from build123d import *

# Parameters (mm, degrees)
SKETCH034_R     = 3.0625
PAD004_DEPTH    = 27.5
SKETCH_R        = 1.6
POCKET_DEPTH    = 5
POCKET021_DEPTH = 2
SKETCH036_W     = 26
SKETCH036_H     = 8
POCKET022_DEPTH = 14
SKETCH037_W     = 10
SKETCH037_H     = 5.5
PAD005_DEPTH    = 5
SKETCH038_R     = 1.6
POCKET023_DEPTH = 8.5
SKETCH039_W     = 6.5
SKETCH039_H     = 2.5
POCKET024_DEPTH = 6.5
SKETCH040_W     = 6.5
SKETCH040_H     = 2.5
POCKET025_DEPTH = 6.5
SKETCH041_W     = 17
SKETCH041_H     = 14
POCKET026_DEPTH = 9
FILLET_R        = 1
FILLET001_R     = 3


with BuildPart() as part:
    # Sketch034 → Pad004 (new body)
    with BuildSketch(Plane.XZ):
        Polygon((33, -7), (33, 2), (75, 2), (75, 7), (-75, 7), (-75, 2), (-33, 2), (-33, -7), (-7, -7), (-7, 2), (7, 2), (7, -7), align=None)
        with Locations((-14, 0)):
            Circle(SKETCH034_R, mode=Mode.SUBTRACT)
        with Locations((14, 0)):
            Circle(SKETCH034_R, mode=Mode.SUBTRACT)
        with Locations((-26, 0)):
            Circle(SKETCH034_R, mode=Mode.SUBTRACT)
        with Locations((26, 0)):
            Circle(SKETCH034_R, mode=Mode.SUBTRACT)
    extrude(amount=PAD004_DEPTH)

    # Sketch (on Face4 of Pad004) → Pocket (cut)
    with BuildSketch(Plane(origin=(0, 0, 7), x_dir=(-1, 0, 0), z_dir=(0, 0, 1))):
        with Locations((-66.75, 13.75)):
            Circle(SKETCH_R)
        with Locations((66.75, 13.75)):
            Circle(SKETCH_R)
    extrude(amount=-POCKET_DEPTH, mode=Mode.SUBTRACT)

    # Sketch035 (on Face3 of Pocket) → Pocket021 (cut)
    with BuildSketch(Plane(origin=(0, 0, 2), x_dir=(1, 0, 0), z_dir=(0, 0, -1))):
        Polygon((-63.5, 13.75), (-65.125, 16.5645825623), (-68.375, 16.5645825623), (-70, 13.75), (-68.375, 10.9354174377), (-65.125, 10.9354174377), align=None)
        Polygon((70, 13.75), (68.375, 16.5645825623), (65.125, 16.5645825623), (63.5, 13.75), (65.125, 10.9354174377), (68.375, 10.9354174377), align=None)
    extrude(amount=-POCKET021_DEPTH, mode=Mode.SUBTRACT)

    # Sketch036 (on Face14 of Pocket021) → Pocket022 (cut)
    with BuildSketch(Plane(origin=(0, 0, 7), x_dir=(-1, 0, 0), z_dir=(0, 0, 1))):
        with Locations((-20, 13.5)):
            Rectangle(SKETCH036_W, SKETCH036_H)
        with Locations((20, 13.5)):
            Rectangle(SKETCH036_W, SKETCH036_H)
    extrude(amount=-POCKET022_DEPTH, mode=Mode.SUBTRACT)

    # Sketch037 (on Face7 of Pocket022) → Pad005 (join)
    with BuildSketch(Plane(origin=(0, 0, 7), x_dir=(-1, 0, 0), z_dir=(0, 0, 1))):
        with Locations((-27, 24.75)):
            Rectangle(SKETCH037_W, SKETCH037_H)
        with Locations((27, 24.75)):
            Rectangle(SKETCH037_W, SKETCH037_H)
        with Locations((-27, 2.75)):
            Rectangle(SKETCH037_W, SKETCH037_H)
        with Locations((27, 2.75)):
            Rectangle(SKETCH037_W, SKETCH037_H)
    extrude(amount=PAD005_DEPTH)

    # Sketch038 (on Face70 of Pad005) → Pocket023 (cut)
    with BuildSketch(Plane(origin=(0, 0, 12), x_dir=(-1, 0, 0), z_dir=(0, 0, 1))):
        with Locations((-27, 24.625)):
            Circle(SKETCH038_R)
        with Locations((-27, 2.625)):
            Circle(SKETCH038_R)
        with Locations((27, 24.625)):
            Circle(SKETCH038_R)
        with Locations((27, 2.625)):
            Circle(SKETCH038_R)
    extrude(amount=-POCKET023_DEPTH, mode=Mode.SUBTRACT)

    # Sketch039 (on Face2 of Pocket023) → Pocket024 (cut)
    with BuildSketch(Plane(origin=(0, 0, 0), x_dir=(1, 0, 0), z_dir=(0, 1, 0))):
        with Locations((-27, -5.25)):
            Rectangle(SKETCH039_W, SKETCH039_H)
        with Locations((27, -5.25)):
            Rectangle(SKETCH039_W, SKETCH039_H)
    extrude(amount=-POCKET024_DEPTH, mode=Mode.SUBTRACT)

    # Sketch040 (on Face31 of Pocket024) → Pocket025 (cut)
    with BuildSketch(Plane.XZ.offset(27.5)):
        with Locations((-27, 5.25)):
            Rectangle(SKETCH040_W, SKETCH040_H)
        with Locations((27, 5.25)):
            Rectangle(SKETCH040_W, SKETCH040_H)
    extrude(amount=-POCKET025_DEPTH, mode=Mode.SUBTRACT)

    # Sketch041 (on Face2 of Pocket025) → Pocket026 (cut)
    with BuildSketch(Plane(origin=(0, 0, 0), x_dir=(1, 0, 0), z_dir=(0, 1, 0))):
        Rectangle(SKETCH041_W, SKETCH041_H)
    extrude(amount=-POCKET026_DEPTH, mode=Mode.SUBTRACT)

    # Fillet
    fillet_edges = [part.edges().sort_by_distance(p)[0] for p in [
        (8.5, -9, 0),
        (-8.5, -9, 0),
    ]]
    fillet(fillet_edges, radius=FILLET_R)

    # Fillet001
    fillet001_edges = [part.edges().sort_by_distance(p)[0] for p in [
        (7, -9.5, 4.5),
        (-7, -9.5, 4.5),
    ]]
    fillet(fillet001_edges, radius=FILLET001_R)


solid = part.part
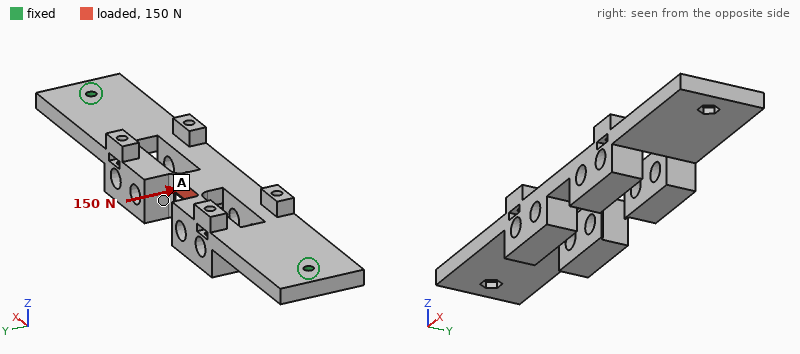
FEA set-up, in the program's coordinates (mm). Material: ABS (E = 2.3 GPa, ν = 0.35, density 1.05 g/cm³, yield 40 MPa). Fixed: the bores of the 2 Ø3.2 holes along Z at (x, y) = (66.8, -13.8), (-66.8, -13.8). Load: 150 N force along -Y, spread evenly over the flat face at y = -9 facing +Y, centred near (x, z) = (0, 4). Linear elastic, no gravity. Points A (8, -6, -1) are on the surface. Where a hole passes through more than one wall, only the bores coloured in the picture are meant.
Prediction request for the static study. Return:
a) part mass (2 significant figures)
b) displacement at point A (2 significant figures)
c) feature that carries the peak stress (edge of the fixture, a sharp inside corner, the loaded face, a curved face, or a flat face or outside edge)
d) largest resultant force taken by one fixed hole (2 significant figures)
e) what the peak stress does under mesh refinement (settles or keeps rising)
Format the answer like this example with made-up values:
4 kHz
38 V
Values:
26 g
0.93 mm
edge of the fixture
180 N
keeps rising
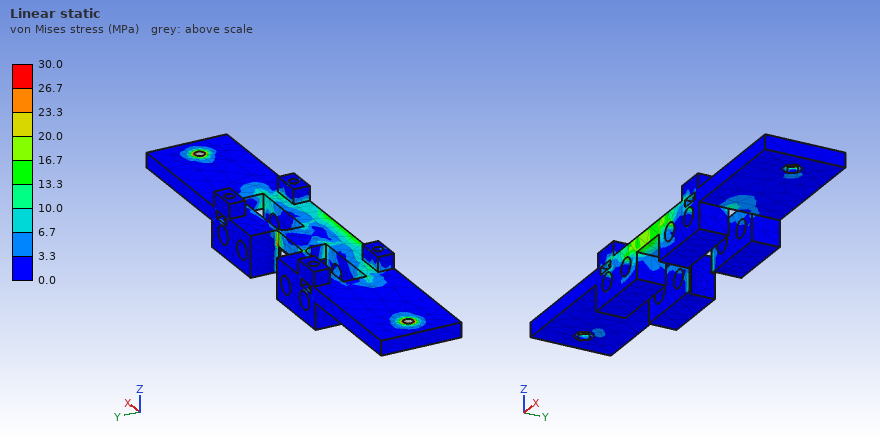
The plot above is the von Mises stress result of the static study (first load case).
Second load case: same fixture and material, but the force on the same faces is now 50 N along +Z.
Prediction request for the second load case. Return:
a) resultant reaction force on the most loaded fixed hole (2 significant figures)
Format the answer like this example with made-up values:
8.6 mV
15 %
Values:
45 N
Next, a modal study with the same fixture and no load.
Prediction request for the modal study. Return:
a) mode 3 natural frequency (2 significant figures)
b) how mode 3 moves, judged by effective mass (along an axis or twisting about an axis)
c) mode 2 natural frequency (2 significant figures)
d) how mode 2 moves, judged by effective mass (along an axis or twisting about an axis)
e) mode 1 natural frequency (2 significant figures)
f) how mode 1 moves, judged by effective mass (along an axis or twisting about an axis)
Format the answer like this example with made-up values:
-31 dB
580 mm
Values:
780 Hz
along Y
580 Hz
along Y
300 Hz
along Z
